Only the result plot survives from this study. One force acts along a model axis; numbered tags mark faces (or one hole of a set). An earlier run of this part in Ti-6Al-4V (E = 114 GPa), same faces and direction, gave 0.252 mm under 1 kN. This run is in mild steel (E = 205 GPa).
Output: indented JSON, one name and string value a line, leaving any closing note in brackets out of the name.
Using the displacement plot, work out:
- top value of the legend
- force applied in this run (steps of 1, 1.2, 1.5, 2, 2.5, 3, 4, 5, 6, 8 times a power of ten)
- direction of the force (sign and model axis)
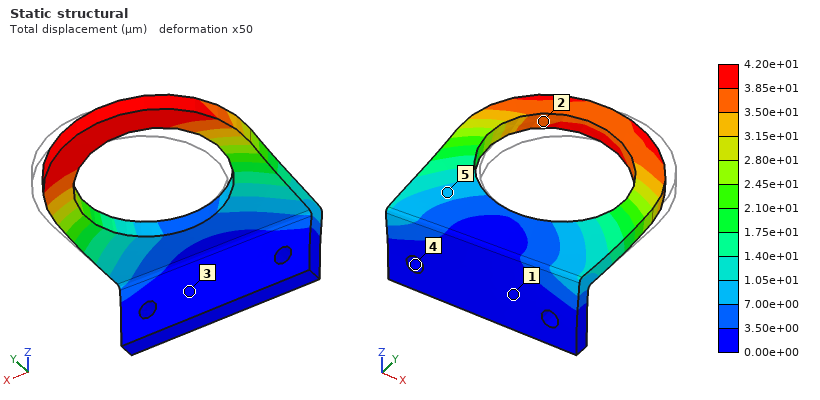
{
  "top value of the legend": "4.20e+01 µm",
  "force applied in this run": "300 N",
  "direction of the force": "-X"
}
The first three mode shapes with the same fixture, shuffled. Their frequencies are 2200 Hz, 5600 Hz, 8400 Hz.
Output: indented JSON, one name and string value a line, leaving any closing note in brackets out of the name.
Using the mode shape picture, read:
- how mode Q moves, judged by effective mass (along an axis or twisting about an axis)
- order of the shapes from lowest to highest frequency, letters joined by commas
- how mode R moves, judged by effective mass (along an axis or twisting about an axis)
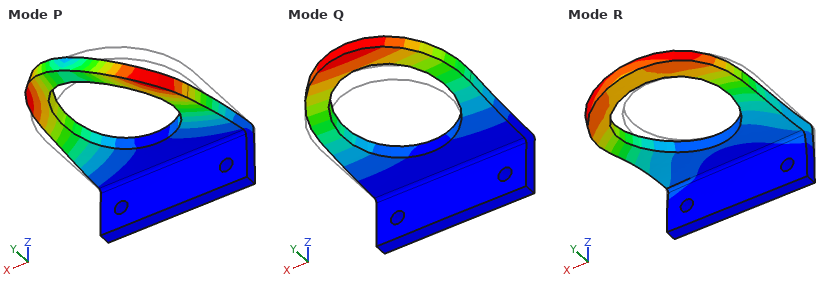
{
  "how mode Q moves, judged by effective mass": "along Z",
  "order of the shapes from lowest to highest frequency, letters joined by commas": "Q, P, R",
  "how mode R moves, judged by effective mass": "along X"
}
